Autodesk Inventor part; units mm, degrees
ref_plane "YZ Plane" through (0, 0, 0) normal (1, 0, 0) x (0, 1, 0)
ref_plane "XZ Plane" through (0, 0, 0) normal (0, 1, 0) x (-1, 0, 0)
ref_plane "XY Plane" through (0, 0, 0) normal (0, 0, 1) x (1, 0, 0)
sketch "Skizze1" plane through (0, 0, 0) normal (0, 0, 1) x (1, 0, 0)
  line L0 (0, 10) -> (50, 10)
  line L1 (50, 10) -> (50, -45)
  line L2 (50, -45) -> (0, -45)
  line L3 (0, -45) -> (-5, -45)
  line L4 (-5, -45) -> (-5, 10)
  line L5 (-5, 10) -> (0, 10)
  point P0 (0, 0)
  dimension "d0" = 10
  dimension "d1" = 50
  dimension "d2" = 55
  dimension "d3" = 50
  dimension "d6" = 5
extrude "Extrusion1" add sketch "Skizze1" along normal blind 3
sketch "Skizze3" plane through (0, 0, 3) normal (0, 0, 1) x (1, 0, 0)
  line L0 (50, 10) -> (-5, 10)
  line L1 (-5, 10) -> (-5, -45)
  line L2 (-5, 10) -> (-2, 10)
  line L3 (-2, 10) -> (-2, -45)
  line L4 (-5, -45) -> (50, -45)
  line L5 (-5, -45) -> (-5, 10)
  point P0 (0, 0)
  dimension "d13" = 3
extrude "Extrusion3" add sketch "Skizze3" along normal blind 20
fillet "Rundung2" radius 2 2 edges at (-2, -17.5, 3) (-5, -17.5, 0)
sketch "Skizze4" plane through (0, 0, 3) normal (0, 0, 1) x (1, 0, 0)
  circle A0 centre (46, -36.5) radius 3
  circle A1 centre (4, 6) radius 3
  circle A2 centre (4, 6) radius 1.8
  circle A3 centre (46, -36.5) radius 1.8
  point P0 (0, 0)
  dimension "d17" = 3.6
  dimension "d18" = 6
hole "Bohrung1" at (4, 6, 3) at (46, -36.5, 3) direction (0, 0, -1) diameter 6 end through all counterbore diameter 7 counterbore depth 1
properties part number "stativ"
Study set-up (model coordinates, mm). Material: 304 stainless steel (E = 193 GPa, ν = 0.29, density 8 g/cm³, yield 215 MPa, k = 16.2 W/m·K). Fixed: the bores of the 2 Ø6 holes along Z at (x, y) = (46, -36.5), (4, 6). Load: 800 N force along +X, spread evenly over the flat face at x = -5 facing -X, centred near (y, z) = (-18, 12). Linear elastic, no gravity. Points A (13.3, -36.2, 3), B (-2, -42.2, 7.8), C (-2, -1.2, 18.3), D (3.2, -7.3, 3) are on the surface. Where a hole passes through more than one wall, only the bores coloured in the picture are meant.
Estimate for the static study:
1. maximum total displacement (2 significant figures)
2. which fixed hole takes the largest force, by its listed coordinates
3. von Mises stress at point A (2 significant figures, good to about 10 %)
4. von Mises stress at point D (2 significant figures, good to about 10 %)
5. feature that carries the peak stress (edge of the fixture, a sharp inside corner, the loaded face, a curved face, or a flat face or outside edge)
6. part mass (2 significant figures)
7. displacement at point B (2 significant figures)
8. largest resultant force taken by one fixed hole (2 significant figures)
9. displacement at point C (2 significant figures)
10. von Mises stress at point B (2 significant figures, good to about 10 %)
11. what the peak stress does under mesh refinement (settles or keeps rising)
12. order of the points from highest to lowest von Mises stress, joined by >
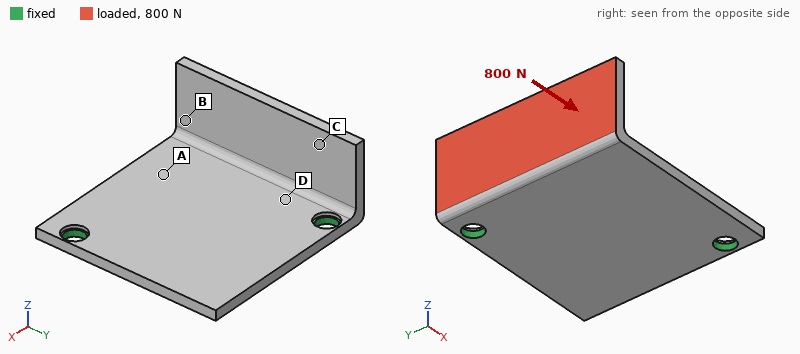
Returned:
0.21 mm
(46, -36.5)
57 MPa
90 MPa
edge of the fixture
97 g
0.11 mm
460 N
0.10 mm
36 MPa
keeps rising
D > A > B > C
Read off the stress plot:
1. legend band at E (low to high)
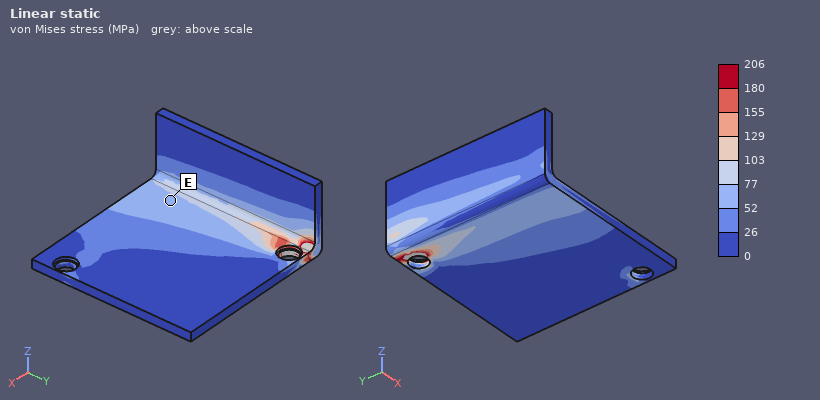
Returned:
52 to 77 MPa
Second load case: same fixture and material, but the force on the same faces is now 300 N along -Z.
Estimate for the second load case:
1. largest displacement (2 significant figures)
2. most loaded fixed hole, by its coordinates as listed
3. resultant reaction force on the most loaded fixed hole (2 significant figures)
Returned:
0.16 mm
(4, 6)
270 N
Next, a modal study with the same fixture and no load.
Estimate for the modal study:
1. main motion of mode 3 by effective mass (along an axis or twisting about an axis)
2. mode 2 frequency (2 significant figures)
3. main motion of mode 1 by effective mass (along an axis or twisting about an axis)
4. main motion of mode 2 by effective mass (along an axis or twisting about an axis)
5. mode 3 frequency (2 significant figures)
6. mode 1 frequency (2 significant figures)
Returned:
along X
2300 Hz
along Z
along Z
3000 Hz
1300 Hz
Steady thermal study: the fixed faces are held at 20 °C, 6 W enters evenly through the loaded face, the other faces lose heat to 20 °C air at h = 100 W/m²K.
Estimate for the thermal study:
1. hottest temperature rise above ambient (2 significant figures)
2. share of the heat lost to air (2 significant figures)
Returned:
24 K
80 %
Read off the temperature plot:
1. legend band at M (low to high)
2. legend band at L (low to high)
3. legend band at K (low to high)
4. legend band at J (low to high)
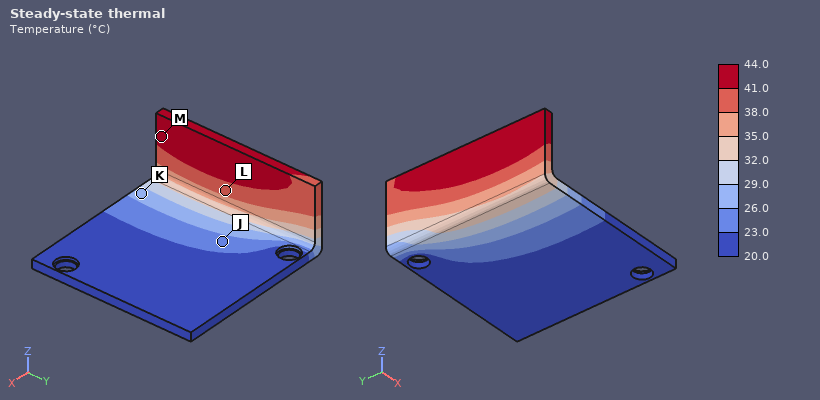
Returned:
41.0 to 44.0 °C
38.0 to 41.0 °C
26.0 to 29.0 °C
23.0 to 26.0 °C
